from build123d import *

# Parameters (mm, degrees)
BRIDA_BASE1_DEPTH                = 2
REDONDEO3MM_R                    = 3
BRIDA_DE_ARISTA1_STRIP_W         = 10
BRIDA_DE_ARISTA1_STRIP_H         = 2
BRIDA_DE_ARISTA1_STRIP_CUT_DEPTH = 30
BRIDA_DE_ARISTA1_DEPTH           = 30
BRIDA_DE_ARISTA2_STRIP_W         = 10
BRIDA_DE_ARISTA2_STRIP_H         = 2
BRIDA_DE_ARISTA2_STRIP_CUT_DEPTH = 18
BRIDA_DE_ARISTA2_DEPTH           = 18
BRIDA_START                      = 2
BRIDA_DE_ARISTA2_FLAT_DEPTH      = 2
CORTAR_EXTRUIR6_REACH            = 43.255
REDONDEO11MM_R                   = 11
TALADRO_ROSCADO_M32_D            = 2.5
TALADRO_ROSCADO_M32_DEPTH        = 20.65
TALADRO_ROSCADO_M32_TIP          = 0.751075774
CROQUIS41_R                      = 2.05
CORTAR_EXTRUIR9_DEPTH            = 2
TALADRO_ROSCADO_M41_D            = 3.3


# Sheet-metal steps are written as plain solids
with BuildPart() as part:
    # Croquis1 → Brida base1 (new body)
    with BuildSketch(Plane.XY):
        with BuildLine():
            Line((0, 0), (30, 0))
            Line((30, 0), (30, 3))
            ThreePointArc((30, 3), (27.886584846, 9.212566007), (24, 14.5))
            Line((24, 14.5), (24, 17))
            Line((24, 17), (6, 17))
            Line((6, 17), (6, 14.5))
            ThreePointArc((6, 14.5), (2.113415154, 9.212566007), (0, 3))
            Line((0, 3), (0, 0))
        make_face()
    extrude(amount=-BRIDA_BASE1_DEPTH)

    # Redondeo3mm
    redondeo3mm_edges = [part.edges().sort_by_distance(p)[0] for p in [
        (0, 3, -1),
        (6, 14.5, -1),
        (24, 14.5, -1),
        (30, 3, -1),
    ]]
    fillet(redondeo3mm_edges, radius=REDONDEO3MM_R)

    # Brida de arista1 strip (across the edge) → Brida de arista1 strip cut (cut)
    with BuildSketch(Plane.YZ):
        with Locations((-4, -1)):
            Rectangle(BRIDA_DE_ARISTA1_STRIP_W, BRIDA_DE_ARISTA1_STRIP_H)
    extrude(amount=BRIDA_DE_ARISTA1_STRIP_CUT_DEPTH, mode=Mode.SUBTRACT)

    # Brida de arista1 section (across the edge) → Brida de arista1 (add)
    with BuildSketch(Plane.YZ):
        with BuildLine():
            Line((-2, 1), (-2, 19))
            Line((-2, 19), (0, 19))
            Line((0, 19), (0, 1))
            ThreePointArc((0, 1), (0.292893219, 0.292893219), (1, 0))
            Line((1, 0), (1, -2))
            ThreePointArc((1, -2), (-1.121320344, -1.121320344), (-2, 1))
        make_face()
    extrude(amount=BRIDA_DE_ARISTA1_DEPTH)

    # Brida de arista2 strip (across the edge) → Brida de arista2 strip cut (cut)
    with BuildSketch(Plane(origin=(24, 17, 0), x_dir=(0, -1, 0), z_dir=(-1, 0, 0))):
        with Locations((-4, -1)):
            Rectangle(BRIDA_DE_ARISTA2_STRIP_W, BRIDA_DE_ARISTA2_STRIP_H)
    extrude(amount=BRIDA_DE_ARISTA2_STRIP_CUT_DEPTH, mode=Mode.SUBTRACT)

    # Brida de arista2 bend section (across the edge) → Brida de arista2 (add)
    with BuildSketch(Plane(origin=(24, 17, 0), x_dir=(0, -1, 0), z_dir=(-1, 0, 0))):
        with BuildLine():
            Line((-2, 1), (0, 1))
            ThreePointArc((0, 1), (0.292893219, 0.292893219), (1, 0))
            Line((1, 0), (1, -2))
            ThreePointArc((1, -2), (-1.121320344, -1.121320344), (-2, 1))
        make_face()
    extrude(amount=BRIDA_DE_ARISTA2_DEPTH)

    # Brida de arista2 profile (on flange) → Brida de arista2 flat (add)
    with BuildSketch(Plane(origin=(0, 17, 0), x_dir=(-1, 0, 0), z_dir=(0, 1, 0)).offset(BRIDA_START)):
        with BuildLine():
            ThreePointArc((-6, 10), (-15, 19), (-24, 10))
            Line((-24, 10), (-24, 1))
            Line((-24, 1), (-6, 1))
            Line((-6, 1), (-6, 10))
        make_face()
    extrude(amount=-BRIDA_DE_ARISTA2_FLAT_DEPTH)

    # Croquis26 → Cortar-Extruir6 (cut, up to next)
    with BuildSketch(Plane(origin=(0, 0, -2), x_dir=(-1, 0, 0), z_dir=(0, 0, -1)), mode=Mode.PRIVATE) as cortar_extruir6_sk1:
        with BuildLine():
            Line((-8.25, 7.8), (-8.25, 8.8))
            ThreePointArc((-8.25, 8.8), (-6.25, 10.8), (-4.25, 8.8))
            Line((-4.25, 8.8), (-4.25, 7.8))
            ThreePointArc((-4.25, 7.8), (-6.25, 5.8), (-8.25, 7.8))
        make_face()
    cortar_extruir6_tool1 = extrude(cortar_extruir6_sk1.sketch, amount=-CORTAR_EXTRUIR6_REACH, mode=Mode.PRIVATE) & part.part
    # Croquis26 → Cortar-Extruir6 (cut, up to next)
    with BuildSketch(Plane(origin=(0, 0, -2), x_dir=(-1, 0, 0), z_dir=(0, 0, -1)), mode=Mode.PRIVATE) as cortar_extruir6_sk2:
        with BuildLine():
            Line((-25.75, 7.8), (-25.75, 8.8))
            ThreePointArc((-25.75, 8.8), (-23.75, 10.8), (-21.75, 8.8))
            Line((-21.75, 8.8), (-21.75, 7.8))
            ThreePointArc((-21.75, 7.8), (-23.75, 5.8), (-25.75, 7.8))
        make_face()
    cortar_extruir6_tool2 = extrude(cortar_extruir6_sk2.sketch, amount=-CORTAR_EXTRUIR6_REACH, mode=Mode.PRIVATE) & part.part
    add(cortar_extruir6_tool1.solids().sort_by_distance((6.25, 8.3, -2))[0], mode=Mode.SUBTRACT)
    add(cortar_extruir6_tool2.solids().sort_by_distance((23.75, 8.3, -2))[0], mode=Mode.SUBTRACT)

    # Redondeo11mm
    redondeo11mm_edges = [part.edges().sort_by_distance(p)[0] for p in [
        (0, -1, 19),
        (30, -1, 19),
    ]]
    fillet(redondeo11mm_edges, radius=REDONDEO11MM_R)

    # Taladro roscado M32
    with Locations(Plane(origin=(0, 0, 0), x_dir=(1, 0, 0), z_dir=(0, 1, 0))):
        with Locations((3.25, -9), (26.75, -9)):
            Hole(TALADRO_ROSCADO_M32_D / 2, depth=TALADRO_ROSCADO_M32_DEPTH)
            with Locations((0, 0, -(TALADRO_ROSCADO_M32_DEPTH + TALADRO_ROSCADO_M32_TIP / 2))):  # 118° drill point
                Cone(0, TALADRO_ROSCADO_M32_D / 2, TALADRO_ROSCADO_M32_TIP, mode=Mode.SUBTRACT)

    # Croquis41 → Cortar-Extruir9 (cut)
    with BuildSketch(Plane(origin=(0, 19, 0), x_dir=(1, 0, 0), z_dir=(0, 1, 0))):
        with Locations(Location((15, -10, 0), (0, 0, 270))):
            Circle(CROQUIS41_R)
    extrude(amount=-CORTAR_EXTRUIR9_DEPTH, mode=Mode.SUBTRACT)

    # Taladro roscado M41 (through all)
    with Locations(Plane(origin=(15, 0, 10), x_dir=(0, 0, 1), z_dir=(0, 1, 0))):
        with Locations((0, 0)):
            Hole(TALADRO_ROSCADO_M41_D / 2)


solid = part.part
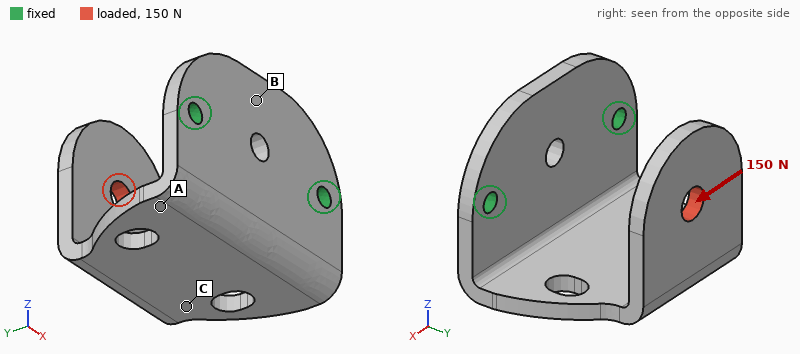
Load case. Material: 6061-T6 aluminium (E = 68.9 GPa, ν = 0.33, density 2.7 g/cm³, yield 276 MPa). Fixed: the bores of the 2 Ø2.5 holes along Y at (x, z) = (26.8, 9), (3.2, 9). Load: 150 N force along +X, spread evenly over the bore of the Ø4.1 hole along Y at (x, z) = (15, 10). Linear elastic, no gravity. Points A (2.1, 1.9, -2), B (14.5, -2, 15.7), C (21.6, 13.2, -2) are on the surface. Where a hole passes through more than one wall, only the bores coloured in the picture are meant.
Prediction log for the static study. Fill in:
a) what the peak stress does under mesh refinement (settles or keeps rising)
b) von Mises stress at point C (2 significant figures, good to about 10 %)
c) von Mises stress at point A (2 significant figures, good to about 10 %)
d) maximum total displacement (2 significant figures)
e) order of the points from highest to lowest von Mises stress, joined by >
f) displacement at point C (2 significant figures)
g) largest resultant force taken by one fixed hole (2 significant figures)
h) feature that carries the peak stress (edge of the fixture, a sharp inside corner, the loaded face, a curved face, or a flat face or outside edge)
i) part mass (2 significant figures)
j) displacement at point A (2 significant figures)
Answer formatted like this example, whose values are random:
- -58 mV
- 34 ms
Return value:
- keeps rising
- 92 MPa
- 45 MPa
- 0.49 mm
- C > A > B
- 0.12 mm
- 140 N
- edge of the fixture
- 6.7 g
- 0.087 mm
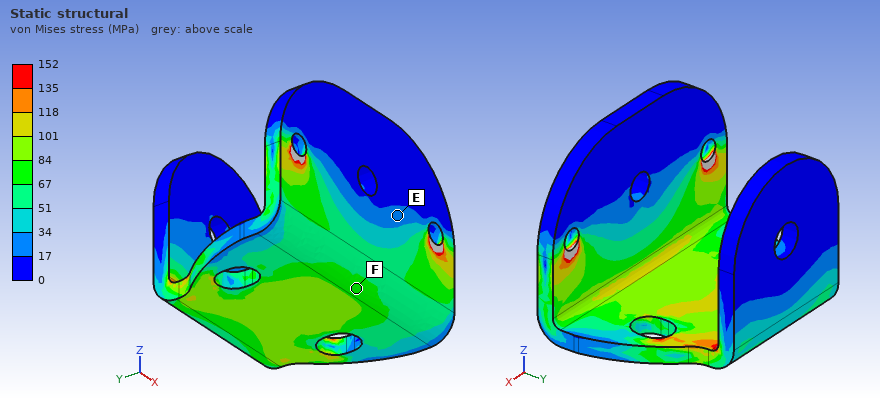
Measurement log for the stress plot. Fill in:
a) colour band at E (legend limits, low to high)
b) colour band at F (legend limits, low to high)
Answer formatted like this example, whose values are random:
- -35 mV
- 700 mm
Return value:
- 17 to 34 MPa
- 67 to 84 MPa
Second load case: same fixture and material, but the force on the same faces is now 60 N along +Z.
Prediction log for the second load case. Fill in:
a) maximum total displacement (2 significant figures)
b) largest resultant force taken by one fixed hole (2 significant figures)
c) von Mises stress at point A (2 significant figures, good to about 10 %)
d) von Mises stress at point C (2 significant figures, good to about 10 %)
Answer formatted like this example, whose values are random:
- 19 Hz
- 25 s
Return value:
- 0.42 mm
- 31 N
- 39 MPa
- 25 MPa
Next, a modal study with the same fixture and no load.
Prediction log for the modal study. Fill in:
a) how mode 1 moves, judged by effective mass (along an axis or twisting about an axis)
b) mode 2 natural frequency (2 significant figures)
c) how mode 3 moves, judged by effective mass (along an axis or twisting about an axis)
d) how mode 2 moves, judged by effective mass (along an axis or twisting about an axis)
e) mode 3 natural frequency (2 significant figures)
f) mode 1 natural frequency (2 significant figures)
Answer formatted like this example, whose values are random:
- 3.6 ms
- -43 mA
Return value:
- along Z
- 2600 Hz
- along Y
- along X
- 3300 Hz
- 1400 Hz
